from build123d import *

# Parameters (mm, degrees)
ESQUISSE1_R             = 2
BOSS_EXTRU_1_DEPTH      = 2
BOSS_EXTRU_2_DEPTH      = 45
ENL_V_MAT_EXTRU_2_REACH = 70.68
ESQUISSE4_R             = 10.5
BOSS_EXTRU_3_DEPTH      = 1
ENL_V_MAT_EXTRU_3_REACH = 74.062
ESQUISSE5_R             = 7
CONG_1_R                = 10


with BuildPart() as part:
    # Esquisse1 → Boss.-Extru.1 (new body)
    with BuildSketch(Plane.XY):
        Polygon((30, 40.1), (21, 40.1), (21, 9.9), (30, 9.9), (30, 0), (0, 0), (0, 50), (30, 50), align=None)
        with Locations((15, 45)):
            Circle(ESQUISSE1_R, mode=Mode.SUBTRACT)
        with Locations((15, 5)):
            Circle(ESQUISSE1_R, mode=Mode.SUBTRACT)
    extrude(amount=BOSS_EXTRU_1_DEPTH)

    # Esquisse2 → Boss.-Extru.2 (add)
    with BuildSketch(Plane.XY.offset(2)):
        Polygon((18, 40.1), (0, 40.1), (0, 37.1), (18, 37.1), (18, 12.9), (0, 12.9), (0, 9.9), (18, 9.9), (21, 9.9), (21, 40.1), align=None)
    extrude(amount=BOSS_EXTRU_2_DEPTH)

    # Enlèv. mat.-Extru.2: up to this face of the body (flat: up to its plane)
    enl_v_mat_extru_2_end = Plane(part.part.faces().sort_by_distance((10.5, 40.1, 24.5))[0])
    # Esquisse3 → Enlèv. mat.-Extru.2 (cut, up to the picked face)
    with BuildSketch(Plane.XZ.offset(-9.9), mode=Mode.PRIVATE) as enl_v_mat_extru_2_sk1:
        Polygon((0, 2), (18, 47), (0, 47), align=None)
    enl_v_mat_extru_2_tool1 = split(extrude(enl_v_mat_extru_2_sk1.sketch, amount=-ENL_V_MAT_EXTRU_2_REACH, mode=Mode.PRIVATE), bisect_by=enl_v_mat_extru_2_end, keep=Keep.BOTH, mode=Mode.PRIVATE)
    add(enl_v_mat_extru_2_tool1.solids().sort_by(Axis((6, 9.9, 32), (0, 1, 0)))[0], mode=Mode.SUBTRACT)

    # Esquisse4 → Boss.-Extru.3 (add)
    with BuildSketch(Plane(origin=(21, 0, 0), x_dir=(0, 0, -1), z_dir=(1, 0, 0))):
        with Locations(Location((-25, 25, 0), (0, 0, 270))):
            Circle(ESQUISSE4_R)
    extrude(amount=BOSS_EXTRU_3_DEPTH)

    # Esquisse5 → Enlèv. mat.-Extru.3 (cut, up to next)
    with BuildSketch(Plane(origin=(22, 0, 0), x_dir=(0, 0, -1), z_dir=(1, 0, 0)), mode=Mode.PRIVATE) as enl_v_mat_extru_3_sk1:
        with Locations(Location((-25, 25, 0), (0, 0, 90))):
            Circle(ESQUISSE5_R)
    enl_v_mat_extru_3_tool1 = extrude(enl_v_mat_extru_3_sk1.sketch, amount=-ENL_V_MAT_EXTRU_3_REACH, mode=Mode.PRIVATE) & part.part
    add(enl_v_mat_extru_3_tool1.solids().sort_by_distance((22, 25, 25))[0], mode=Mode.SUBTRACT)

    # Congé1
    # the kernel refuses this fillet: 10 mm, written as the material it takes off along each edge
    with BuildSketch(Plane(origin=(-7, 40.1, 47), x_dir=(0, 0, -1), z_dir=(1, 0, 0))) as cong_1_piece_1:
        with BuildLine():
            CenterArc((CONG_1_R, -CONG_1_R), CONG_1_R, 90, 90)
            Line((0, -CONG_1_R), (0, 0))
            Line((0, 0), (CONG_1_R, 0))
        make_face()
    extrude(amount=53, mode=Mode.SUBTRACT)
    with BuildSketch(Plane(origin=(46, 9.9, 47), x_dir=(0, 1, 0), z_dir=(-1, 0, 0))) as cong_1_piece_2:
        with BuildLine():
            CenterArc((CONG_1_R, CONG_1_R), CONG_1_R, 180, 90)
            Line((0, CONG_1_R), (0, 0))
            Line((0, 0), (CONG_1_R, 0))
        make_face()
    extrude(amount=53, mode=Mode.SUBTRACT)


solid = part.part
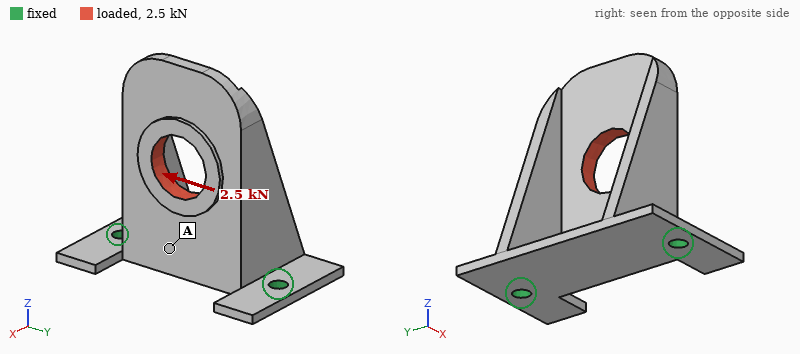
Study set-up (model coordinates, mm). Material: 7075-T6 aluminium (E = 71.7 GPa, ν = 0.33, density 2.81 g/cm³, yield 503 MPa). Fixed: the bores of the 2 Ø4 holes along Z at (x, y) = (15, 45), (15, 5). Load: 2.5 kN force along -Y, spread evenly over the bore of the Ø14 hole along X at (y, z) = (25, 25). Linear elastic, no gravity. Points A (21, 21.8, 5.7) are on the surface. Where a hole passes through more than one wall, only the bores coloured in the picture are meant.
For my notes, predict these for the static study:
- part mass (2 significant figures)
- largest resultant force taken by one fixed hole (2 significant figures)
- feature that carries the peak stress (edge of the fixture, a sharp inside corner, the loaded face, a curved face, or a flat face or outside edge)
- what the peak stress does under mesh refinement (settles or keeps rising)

24 g
2.2 kN
edge of the fixture
keeps rising
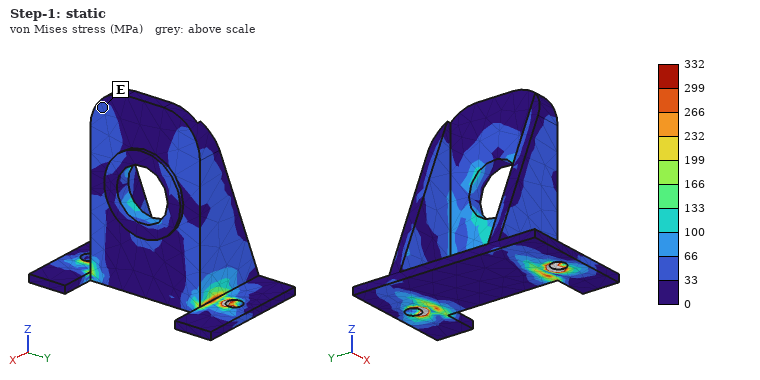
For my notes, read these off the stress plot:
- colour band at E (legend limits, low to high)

33 to 66 MPa
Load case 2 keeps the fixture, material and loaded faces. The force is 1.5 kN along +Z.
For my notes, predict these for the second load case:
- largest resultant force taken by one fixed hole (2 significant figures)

850 N
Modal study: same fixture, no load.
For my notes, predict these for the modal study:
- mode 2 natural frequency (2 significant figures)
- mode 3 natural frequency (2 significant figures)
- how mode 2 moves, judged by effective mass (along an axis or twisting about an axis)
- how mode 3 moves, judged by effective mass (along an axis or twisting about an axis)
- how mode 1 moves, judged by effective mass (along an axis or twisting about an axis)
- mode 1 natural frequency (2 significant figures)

3700 Hz
6100 Hz
along Y
along Y
along X
1400 Hz
